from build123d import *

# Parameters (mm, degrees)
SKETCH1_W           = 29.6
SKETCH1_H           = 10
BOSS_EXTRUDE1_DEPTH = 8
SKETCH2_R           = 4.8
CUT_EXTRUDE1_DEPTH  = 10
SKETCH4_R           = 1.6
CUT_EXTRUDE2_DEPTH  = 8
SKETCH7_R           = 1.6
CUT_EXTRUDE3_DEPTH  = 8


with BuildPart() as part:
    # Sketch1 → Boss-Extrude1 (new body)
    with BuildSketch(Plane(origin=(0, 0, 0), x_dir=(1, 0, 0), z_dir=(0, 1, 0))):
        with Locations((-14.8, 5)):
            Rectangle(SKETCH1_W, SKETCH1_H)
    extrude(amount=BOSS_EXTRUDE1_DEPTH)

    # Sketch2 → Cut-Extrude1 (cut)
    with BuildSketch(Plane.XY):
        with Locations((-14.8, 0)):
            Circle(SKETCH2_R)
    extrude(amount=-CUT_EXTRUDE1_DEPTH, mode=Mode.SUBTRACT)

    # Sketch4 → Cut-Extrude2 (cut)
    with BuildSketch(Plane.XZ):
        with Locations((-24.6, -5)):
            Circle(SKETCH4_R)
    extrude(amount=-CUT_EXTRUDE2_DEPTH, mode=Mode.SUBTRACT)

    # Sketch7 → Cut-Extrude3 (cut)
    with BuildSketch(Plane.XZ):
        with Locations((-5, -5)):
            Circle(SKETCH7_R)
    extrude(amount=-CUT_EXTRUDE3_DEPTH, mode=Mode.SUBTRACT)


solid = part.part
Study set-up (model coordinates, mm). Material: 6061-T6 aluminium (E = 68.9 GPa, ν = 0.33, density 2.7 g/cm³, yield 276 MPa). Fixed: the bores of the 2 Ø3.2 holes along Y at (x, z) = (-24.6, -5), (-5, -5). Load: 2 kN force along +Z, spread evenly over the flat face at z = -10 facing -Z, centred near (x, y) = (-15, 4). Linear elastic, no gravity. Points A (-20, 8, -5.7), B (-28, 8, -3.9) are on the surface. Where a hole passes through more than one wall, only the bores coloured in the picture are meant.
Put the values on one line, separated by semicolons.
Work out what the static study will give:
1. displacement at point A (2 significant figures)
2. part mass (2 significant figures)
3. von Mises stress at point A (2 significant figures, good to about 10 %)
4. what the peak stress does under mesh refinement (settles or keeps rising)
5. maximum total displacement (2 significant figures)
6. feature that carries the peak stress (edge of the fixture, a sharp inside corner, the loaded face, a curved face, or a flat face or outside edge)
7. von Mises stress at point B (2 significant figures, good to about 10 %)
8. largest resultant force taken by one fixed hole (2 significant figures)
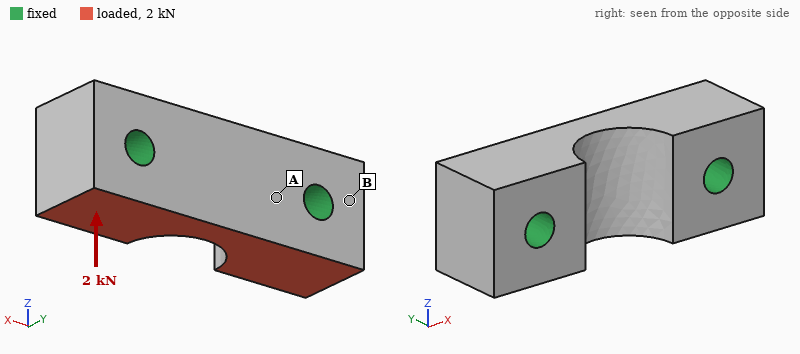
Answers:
1.7 µm; 5.1 g; 14 MPa; keeps rising; 3.3 µm; edge of the fixture; 5.5 MPa; 1.0 kN
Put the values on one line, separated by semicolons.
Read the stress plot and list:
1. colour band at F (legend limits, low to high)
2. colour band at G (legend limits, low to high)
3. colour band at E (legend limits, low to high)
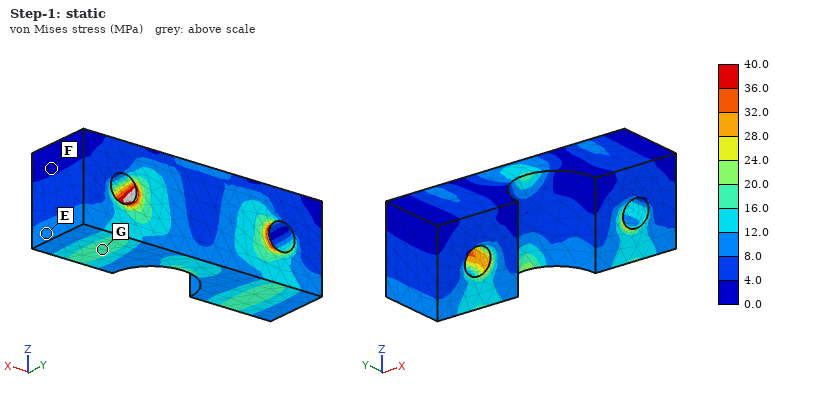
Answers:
0.0 to 4.0 MPa; 16.0 to 20.0 MPa; 8.0 to 12.0 MPa
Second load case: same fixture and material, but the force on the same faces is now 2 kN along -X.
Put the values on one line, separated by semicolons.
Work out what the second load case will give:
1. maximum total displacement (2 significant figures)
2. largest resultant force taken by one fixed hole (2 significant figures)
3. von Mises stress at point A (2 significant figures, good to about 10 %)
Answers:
4.8 µm; 1.0 kN; 14 MPa
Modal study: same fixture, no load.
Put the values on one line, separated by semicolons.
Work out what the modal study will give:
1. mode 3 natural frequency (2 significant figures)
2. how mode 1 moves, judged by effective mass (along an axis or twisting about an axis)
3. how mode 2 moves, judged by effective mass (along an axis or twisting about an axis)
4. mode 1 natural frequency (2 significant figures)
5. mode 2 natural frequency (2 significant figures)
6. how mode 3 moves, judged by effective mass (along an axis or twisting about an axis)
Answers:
92 kHz; along Z; along Y; 62 kHz; 73 kHz; twisting about X
